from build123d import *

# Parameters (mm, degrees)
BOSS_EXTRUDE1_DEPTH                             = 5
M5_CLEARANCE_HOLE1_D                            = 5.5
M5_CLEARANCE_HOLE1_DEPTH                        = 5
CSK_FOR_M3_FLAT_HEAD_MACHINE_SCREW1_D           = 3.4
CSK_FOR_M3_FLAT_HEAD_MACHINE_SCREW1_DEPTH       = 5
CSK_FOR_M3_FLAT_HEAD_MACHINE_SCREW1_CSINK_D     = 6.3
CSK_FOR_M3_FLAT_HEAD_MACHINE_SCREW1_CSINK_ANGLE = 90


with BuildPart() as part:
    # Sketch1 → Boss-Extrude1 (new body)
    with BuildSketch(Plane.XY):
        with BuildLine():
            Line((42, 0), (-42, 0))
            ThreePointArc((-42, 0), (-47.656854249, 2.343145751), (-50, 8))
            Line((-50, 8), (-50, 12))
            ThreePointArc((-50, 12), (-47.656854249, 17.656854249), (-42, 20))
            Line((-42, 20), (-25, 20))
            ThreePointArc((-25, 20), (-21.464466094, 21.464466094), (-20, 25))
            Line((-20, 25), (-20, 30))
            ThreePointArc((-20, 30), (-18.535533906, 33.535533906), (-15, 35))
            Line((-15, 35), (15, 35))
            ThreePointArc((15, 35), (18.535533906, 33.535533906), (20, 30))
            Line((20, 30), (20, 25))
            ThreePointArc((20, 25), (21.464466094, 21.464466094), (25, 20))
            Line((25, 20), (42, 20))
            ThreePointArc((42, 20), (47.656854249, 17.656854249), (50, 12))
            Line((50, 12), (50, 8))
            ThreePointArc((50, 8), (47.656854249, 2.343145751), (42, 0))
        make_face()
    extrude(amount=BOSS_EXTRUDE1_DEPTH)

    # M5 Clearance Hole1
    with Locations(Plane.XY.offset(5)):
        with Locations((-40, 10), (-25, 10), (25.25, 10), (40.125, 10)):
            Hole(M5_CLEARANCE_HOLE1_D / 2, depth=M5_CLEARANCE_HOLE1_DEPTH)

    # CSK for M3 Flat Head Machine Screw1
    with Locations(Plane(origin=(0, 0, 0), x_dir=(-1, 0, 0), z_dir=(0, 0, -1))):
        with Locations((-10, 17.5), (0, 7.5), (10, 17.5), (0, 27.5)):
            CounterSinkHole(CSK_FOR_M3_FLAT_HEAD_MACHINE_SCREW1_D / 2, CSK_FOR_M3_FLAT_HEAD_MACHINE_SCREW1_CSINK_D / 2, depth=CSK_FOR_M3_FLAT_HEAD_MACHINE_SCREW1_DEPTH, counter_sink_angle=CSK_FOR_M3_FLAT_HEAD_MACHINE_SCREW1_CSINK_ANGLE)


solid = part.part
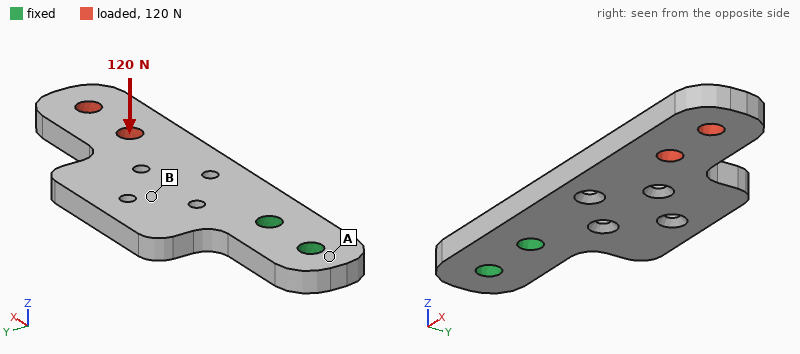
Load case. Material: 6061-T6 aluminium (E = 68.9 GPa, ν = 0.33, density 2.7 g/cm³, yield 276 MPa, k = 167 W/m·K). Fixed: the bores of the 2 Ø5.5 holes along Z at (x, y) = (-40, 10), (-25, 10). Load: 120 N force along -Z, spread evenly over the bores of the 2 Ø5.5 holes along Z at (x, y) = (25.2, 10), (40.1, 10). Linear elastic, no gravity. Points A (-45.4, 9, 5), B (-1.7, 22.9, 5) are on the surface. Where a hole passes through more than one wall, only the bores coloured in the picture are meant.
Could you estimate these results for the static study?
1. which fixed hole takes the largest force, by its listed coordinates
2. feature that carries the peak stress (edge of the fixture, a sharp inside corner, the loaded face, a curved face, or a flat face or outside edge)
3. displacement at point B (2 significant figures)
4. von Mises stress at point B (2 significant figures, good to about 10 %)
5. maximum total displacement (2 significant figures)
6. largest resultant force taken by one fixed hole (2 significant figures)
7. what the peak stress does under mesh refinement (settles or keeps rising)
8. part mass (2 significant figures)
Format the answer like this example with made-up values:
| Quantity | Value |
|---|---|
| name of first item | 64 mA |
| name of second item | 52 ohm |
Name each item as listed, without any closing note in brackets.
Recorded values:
| Quantity | Value |
|---|---|
| which fixed hole takes the largest force, by its listed coordinates | (-25, 10) |
| feature that carries the peak stress | edge of the fixture |
| displacement at point B | 0.094 mm |
| von Mises stress at point B | 30 MPa |
| maximum total displacement | 0.61 mm |
| largest resultant force taken by one fixed hole | 210 N |
| what the peak stress does under mesh refinement | keeps rising |
| part mass | 32 g |
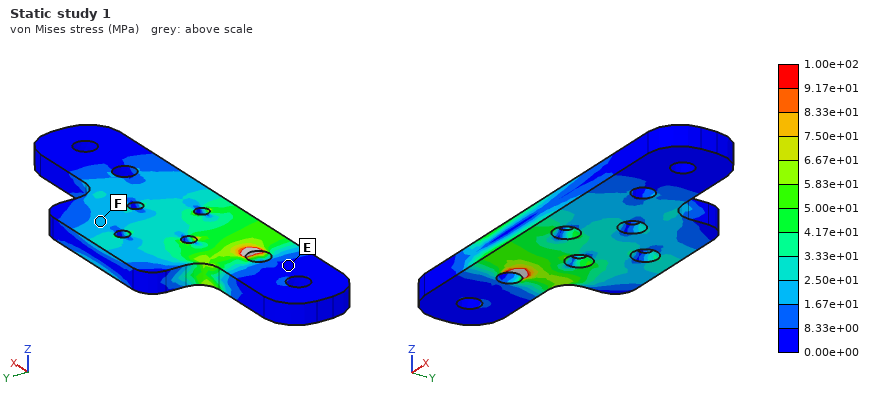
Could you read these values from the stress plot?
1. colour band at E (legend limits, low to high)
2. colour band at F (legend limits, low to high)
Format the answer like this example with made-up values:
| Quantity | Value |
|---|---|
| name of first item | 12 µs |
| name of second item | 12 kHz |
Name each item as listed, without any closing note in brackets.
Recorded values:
| Quantity | Value |
|---|---|
| colour band at E | 0.00e+00 to 8.33e+00 MPa |
| colour band at F | 1.67e+01 to 2.50e+01 MPa |
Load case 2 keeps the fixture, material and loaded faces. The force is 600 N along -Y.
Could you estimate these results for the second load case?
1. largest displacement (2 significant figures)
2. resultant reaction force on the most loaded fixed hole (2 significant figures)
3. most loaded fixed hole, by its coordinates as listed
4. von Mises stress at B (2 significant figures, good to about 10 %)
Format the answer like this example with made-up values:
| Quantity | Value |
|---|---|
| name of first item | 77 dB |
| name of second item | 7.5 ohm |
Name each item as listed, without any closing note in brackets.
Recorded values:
| Quantity | Value |
|---|---|
| largest displacement | 0.24 mm |
| resultant reaction force on the most loaded fixed hole | 1.8 kN |
| most loaded fixed hole, by its coordinates as listed | (-25, 10) |
| von Mises stress at B | 16 MPa |
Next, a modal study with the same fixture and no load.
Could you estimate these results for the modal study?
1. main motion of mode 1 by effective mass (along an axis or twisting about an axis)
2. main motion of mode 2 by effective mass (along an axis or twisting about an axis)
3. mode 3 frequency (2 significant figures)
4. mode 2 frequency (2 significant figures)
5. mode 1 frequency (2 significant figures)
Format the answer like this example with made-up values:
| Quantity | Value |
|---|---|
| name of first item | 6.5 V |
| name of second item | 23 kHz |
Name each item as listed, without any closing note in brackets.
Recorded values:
| Quantity | Value |
|---|---|
| main motion of mode 1 by effective mass | along Z |
| main motion of mode 2 by effective mass | along Y |
| mode 3 frequency | 2900 Hz |
| mode 2 frequency | 2700 Hz |
| mode 1 frequency | 840 Hz |
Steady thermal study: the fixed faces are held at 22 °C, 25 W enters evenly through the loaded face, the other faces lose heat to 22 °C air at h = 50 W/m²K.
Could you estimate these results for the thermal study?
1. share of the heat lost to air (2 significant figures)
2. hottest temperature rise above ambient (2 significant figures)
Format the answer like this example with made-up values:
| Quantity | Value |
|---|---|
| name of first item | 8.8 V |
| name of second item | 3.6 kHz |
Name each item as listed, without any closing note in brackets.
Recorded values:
| Quantity | Value |
|---|---|
| share of the heat lost to air | 30 % |
| hottest temperature rise above ambient | 60 K |
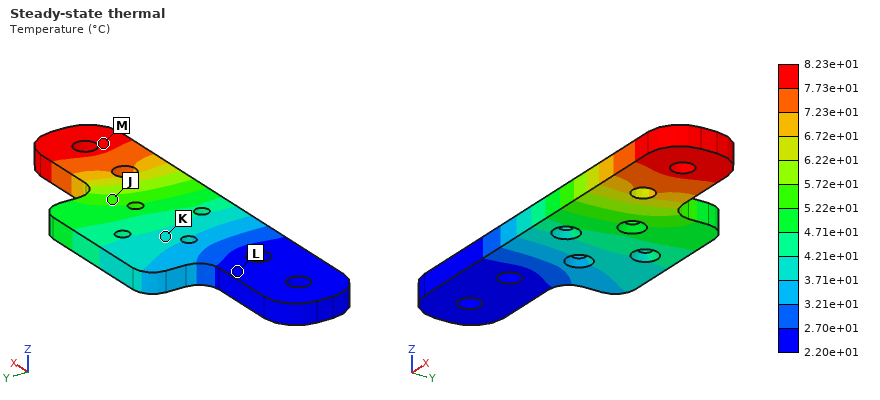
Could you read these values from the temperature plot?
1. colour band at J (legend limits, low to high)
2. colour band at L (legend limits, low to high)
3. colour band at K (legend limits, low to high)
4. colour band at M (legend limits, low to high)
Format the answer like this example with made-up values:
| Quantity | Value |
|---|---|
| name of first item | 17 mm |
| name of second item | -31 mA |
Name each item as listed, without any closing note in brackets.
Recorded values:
| Quantity | Value |
|---|---|
| colour band at J | 5.22e+01 to 5.72e+01 °C |
| colour band at L | 2.20e+01 to 2.70e+01 °C |
| colour band at K | 3.71e+01 to 4.21e+01 °C |
| colour band at M | 7.73e+01 to 8.23e+01 °C |
